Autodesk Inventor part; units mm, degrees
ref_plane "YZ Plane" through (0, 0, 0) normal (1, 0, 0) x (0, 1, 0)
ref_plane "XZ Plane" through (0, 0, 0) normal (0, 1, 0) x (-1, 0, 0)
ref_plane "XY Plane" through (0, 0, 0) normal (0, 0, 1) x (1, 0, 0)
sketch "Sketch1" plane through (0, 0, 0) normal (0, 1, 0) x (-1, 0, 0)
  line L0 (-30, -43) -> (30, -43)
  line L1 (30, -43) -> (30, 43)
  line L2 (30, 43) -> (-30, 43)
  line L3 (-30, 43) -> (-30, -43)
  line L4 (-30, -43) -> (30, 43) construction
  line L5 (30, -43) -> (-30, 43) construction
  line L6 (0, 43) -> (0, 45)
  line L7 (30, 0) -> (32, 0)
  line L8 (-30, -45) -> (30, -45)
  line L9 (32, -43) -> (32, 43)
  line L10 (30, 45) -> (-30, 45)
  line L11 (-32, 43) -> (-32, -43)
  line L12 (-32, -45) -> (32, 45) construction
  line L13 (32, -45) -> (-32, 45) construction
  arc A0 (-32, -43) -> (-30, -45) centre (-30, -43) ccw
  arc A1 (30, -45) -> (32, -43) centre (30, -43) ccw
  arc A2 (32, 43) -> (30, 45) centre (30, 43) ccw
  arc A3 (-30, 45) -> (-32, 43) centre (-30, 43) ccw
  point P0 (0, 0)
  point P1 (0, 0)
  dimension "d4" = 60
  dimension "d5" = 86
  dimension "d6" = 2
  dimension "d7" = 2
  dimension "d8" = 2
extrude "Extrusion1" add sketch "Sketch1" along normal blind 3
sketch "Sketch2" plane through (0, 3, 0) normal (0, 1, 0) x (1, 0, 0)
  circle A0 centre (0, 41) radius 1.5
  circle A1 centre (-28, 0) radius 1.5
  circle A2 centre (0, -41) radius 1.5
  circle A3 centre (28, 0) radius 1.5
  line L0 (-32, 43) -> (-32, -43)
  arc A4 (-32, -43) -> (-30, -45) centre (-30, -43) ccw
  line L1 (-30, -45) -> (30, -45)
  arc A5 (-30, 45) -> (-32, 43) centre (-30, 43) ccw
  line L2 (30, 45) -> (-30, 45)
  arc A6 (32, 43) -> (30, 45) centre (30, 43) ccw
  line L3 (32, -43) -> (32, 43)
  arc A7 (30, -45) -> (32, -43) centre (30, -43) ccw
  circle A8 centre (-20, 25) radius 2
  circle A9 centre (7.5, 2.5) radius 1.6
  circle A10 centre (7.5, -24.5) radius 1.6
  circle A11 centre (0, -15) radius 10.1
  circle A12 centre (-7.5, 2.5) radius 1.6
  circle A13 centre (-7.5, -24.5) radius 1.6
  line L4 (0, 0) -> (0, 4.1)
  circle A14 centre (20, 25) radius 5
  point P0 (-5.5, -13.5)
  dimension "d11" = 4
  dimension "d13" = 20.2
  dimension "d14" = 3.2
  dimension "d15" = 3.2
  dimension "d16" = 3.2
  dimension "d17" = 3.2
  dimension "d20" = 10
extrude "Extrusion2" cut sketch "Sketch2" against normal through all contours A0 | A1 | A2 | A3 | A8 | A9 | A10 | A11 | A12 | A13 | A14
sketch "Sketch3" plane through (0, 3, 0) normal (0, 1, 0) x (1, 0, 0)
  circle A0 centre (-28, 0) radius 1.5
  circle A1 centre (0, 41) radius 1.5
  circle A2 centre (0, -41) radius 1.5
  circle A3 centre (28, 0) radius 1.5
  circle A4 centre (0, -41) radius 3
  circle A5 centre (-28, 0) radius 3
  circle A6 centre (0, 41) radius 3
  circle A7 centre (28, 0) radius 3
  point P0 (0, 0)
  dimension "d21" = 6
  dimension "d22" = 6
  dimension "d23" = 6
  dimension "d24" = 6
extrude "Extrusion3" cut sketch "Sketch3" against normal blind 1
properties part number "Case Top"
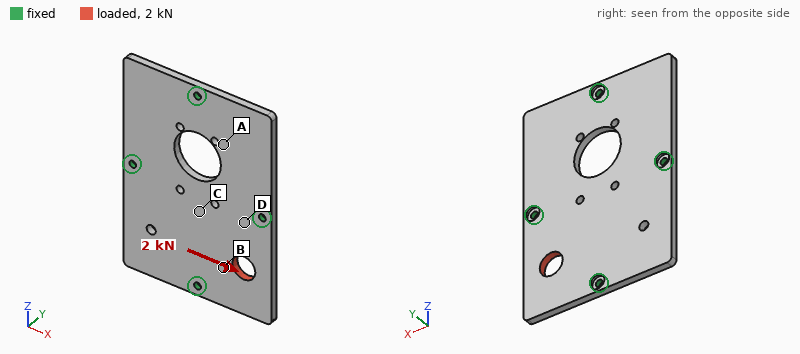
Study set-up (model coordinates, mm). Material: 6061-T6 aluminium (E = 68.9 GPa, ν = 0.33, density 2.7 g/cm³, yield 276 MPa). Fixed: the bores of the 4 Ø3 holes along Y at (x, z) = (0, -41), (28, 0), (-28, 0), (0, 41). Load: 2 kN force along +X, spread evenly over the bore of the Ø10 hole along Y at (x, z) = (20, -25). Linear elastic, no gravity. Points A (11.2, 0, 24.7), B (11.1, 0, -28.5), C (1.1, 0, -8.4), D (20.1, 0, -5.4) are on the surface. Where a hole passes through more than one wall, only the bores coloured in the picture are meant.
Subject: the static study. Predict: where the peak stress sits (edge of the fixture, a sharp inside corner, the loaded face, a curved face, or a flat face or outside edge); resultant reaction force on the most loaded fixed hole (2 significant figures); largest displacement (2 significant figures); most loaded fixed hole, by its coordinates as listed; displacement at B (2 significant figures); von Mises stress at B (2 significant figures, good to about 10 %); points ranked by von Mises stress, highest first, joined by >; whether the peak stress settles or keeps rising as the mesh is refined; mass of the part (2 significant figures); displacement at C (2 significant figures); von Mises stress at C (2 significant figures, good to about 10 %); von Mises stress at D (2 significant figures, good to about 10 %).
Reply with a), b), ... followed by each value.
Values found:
a) edge of the fixture
b) 1.0 kN
c) 16 µm
d) (0, -41)
e) 8.0 µm
f) 22 MPa
g) B > D > C > A
h) keeps rising
i) 43 g
j) 4.7 µm
k) 9.5 MPa
l) 14 MPa
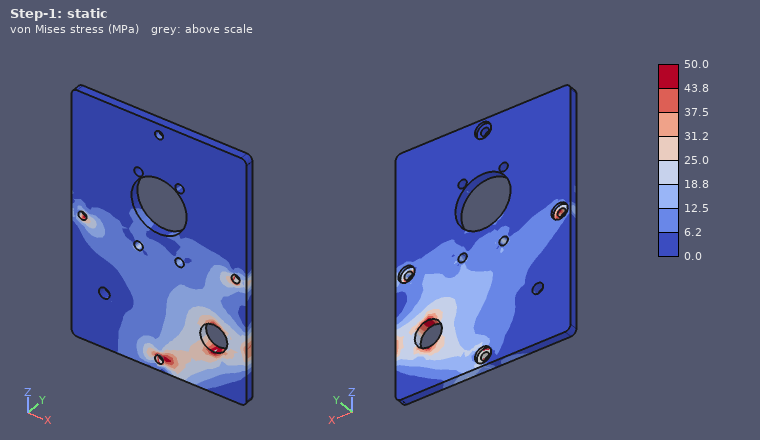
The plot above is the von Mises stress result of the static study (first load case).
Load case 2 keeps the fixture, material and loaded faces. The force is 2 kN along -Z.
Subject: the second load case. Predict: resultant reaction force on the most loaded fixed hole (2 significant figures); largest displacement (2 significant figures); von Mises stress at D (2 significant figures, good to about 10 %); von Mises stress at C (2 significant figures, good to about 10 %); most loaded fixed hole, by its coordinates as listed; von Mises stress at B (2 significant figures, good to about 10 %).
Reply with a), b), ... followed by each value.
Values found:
a) 1.0 kN
b) 14 µm
c) 17 MPa
d) 7.1 MPa
e) (28, 0)
f) 17 MPa
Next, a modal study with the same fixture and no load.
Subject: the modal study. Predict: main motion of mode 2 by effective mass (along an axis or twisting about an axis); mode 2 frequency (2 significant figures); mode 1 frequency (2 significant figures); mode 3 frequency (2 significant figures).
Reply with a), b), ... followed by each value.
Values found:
a) twisting about Z
b) 2900 Hz
c) 2700 Hz
d) 3200 Hz
